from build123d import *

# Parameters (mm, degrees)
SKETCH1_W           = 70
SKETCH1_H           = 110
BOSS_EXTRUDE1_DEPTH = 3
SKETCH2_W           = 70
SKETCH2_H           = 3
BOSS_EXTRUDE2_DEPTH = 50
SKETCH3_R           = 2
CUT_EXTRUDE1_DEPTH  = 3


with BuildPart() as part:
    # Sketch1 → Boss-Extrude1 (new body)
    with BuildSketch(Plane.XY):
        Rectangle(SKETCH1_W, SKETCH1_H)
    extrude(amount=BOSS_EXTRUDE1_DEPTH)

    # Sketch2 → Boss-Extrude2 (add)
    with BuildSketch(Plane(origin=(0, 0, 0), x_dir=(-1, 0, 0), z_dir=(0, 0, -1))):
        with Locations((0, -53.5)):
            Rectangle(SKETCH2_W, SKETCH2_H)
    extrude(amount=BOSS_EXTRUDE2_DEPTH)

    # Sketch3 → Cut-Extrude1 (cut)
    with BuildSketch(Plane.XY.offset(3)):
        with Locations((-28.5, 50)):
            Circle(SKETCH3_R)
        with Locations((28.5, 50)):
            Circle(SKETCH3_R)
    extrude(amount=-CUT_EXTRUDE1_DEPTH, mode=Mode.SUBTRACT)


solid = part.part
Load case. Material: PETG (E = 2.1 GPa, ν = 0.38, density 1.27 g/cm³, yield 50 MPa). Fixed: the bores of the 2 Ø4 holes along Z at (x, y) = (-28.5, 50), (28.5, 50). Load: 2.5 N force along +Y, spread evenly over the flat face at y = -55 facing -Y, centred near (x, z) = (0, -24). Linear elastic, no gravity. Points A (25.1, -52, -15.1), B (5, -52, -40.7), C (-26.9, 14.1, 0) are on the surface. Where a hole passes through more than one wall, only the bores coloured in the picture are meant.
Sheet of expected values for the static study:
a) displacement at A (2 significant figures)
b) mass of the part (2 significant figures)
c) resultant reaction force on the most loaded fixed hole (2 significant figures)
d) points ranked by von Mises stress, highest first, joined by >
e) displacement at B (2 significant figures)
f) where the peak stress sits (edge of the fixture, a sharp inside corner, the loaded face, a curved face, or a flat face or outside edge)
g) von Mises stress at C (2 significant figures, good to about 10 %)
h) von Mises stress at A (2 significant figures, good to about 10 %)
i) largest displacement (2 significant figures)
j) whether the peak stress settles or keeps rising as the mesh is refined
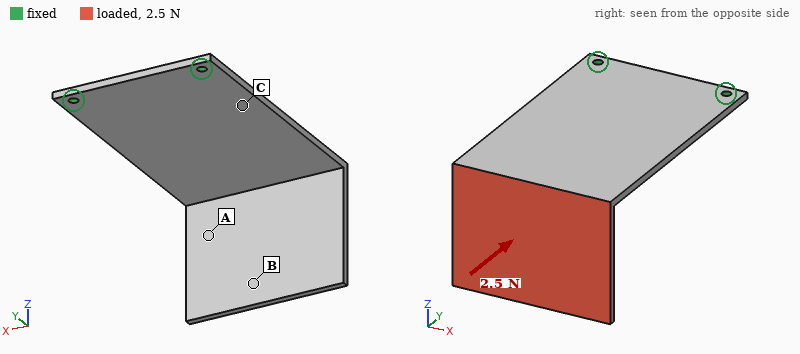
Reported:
1.1 mm
43 g
1.3 N
C > A > B
1.4 mm
edge of the fixture
0.61 MPa
0.24 MPa
1.6 mm
keeps rising
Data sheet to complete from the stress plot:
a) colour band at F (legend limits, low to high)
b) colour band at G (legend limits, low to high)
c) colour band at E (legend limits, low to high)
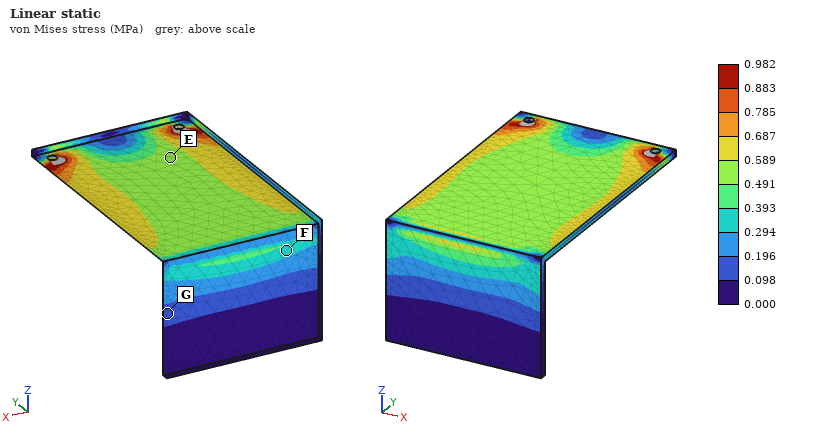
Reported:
0.294 to 0.393 MPa
0.098 to 0.196 MPa
0.491 to 0.589 MPa
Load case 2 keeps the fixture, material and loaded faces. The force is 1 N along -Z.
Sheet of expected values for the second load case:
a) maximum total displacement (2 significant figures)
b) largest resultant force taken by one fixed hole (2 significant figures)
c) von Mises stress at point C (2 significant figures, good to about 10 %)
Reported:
1.7 mm
0.50 N
0.67 MPa
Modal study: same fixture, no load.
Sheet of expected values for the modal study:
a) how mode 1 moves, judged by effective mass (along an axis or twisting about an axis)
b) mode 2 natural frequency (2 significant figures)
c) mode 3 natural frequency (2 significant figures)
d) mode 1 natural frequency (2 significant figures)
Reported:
along Z
85 Hz
130 Hz
29 Hz
